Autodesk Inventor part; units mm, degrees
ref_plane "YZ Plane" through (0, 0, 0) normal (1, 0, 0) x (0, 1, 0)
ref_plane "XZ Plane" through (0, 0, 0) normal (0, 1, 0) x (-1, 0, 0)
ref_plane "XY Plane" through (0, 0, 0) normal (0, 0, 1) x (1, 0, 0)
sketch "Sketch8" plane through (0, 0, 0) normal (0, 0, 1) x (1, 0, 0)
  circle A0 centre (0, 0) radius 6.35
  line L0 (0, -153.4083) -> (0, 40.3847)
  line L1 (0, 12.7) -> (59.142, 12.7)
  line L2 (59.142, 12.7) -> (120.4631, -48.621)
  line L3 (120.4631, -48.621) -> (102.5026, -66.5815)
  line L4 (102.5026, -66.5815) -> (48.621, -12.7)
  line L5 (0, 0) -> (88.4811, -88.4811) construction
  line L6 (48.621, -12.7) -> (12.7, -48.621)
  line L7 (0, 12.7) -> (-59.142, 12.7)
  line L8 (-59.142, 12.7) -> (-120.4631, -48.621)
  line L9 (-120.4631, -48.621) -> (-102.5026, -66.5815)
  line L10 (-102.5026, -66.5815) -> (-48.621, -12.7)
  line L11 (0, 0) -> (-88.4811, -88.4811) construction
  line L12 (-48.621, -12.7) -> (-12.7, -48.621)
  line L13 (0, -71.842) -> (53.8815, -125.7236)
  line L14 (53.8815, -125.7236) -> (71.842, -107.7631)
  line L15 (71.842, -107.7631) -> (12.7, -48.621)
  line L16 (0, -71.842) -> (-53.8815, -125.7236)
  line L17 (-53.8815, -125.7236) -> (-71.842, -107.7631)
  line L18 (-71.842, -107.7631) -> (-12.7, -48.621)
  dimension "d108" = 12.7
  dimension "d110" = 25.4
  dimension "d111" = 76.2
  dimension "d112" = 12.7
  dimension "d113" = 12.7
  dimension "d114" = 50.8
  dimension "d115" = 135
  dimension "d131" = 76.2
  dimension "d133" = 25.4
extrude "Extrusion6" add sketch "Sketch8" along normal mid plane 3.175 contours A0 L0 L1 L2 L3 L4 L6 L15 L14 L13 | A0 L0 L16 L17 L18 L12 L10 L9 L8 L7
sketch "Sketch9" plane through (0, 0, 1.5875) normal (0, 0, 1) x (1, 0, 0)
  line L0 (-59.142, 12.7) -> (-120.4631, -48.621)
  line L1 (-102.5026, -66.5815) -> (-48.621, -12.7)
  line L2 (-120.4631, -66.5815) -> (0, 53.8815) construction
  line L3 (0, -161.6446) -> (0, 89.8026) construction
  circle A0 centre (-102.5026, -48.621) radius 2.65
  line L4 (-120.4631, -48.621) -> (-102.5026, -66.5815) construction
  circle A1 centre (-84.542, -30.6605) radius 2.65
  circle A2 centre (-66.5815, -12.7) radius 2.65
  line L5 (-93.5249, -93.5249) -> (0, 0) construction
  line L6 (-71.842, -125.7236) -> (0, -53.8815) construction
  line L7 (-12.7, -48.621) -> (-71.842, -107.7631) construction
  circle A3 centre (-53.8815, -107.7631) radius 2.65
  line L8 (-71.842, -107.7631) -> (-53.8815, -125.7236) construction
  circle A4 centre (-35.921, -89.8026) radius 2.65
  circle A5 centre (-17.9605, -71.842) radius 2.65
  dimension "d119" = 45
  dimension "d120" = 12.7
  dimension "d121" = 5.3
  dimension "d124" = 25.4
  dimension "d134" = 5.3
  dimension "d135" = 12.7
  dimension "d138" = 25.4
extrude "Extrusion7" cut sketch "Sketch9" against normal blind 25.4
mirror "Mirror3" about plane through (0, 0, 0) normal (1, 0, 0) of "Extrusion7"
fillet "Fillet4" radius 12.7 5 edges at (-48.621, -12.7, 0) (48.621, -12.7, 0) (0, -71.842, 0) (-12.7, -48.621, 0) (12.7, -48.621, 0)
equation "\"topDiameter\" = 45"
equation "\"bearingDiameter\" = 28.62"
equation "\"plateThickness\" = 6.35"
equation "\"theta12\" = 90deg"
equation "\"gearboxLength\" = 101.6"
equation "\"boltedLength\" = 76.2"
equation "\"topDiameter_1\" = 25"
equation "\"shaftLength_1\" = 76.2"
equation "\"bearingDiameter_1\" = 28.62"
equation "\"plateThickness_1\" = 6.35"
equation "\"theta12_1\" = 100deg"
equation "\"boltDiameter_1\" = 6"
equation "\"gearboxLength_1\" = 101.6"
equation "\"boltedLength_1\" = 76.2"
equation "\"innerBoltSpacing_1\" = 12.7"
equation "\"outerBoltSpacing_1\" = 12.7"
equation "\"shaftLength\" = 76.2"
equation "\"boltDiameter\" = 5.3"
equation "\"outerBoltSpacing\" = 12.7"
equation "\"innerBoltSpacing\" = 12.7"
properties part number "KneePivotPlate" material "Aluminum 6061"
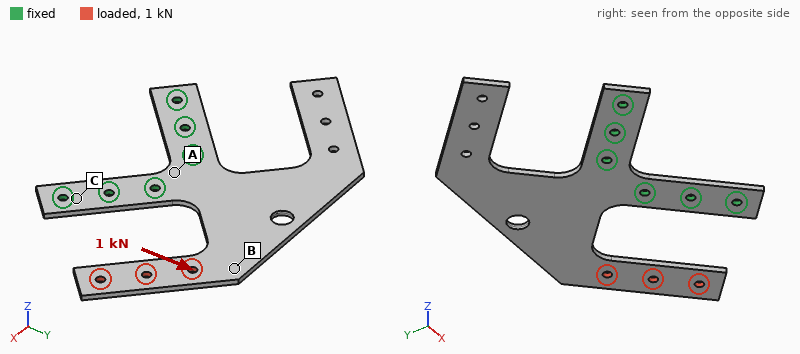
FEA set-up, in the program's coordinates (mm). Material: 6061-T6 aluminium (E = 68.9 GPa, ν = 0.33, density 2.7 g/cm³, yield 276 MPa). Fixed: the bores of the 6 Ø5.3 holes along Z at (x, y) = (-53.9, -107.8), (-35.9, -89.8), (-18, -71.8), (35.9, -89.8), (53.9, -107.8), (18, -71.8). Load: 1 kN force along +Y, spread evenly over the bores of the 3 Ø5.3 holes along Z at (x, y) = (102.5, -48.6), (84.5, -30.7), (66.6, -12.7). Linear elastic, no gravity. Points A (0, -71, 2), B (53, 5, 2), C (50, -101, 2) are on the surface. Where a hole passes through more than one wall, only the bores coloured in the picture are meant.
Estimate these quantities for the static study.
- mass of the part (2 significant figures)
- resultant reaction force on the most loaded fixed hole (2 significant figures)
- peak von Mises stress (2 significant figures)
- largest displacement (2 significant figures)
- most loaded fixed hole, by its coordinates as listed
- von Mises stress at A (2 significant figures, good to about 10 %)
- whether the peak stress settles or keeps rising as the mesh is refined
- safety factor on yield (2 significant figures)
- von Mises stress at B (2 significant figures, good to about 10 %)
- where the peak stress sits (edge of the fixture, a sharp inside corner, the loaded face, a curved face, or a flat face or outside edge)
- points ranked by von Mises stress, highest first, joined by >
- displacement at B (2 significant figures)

110 g
2.4 kN
190 MPa
0.80 mm
(18, -71.8)
26 MPa
settles
1.5
45 MPa
a curved face
B > A > C
0.32 mm
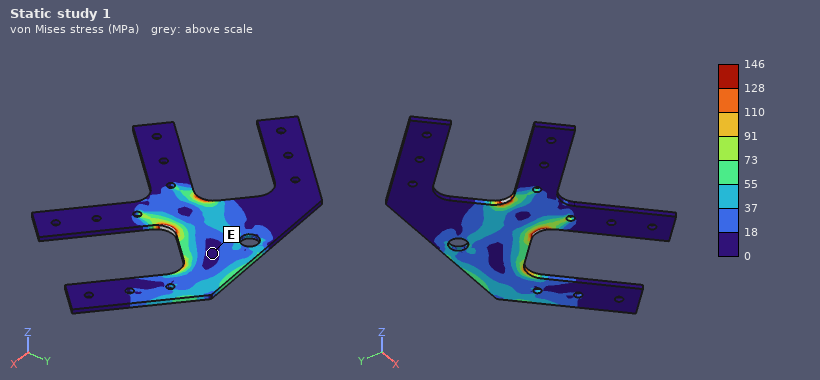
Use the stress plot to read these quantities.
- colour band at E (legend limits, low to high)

0 to 18 MPa
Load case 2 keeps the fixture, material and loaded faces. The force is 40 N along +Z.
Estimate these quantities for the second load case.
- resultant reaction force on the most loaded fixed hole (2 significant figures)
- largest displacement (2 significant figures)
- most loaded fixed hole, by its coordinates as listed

130 N
3.1 mm
(18, -71.8)
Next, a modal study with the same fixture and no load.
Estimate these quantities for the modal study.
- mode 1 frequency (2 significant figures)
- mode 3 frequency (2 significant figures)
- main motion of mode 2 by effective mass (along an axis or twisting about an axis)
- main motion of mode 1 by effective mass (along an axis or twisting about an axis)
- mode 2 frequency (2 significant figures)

150 Hz
240 Hz
along Z
twisting about Y
190 Hz
